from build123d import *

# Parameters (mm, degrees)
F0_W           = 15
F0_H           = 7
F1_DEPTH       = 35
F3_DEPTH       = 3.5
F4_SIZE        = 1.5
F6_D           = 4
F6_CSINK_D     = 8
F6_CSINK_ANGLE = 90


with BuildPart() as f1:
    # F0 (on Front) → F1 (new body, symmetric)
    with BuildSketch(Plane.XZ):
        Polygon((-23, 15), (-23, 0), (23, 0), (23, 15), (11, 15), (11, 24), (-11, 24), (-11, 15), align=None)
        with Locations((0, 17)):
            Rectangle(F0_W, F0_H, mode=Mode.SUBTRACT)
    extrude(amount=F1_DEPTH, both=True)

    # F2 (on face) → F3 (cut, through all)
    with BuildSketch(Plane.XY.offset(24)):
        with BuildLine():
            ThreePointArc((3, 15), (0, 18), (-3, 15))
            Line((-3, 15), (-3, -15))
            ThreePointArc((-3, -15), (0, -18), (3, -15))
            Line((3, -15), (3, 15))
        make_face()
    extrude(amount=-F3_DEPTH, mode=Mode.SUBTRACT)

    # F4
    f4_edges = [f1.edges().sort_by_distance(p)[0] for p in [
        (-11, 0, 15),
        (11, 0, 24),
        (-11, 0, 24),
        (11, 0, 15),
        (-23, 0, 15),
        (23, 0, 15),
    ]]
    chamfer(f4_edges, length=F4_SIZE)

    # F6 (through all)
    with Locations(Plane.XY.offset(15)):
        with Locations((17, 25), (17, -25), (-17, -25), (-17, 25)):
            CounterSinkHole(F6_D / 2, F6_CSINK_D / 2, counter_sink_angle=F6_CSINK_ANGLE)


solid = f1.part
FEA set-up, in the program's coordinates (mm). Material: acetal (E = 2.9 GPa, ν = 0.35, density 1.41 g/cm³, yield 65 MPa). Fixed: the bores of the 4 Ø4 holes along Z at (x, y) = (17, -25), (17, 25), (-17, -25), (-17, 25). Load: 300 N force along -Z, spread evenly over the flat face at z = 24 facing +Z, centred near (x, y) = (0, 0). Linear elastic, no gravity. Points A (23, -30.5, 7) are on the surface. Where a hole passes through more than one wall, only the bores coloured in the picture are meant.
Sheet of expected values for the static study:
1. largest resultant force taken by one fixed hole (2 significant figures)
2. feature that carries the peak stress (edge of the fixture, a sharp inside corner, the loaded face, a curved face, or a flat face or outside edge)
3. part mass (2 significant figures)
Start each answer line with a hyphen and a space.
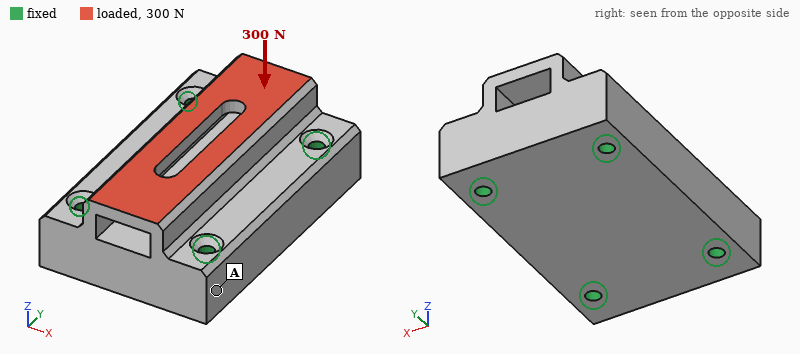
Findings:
- 79 N
- the loaded face
- 75 g
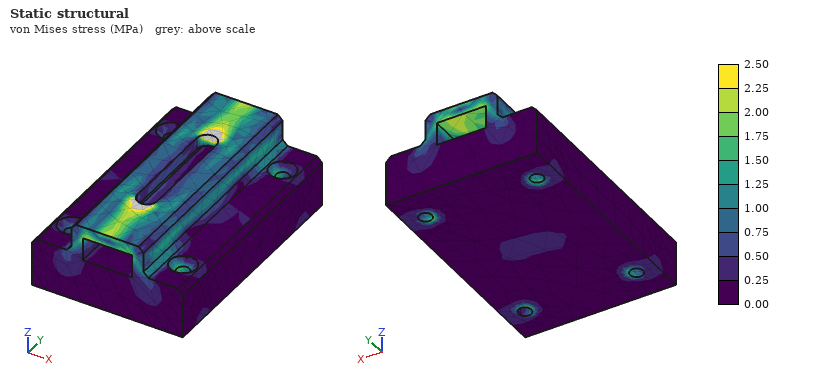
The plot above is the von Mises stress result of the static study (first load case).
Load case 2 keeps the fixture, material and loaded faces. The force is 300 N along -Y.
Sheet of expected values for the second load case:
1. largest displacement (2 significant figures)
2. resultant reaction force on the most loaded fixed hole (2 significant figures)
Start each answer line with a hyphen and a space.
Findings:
- 19 µm
- 88 N
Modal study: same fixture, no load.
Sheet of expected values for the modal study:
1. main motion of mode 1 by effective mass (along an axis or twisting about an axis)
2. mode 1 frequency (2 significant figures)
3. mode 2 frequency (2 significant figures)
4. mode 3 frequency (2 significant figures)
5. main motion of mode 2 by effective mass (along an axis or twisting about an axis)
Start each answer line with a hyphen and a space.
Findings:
- along Z
- 4800 Hz
- 5900 Hz
- 6600 Hz
- along X
